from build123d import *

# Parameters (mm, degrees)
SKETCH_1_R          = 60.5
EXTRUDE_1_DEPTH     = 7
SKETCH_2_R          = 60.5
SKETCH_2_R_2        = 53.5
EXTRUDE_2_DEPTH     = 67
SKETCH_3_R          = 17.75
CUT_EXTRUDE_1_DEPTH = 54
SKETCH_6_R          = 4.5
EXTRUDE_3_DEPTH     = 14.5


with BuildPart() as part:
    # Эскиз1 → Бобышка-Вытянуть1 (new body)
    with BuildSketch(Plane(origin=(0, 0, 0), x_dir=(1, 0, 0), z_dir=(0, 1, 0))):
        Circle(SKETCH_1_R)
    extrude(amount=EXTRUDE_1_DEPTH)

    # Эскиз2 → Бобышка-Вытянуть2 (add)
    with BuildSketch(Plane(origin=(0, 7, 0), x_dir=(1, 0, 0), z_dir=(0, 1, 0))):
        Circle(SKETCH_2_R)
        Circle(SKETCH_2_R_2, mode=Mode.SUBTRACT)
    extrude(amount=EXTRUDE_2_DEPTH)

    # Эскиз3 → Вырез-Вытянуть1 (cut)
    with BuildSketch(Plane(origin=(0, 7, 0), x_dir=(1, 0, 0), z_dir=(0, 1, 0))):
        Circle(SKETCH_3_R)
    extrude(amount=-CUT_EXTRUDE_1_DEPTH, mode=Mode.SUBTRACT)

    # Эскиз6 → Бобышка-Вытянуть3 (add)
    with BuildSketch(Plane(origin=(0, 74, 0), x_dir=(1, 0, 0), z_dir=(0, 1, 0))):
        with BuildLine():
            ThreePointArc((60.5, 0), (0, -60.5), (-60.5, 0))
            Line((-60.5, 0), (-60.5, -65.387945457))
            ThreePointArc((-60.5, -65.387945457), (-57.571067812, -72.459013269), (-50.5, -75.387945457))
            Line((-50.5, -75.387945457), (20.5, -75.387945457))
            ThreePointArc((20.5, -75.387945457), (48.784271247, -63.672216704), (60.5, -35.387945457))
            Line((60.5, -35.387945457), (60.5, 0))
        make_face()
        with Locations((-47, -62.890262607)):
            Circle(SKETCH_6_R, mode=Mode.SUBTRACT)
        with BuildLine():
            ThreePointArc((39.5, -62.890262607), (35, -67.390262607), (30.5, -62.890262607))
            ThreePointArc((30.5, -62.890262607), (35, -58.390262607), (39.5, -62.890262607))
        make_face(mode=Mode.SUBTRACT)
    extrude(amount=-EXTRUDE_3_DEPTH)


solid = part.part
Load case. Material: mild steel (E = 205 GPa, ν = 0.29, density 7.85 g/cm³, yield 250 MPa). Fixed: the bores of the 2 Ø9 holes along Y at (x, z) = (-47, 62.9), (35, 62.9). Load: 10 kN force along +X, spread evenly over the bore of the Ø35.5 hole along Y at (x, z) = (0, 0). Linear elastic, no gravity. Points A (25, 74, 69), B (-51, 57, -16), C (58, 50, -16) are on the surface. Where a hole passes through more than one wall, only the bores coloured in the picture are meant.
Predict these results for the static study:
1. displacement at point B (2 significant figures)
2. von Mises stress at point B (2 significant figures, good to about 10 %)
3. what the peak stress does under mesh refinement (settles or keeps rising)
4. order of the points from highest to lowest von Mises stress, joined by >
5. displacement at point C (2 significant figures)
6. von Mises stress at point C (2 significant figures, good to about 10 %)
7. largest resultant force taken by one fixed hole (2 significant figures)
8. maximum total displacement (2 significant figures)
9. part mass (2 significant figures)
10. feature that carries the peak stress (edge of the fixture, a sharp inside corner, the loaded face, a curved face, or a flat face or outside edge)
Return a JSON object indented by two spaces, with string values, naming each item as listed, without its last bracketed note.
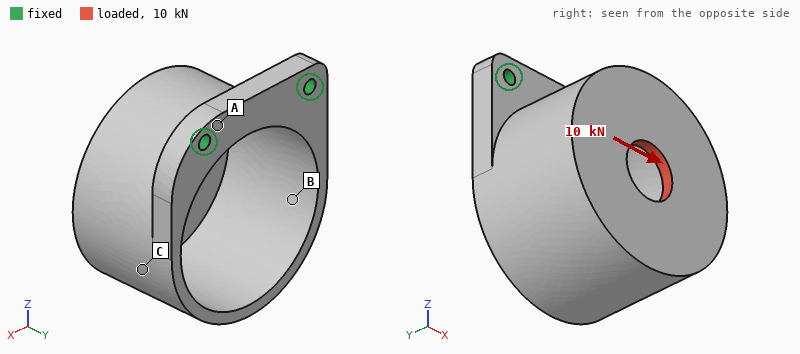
{
  "displacement at point B": "0.13 mm",
  "von Mises stress at point B": "55 MPa",
  "what the peak stress does under mesh refinement": "keeps rising",
  "order of the points from highest to lowest von Mises stress, joined by >": "B > C > A",
  "displacement at point C": "0.14 mm",
  "von Mises stress at point C": "29 MPa",
  "largest resultant force taken by one fixed hole": "11 kN",
  "maximum total displacement": "0.20 mm",
  "part mass": "2.2 kg",
  "feature that carries the peak stress": "edge of the fixture"
}
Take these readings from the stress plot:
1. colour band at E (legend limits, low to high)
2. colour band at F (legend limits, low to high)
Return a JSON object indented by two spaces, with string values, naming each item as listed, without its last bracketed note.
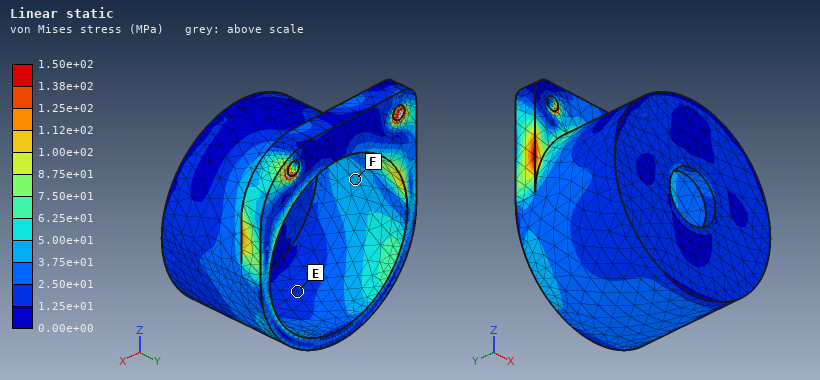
{
  "colour band at E": "1.25e+01 to 2.50e+01 MPa",
  "colour band at F": "3.75e+01 to 5.00e+01 MPa"
}
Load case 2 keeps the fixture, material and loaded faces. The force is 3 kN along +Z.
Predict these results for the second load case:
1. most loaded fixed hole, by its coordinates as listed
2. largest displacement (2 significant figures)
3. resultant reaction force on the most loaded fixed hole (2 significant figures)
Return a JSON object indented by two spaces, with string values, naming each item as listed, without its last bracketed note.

{
  "most loaded fixed hole, by its coordinates as listed": "(35, 62.9)",
  "largest displacement": "0.17 mm",
  "resultant reaction force on the most loaded fixed hole": "1.8 kN"
}
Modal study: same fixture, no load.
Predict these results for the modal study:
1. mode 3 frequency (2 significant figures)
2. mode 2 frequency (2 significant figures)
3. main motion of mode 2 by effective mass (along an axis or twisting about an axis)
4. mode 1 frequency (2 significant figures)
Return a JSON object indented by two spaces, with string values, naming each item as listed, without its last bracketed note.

{
  "mode 3 frequency": "2300 Hz",
  "mode 2 frequency": "890 Hz",
  "main motion of mode 2 by effective mass": "along X",
  "mode 1 frequency": "560 Hz"
}
